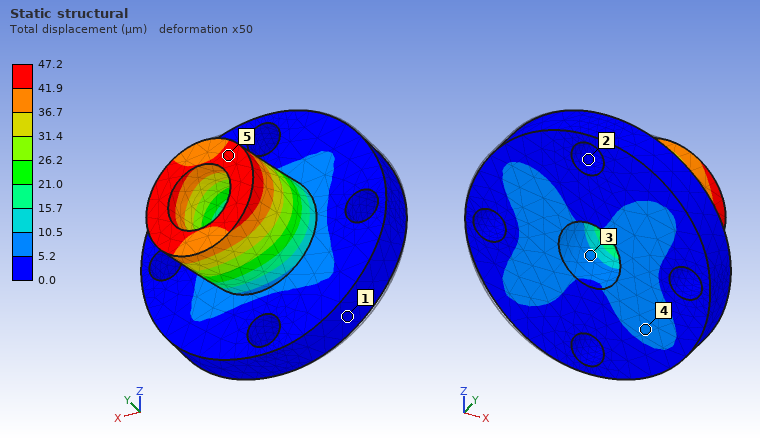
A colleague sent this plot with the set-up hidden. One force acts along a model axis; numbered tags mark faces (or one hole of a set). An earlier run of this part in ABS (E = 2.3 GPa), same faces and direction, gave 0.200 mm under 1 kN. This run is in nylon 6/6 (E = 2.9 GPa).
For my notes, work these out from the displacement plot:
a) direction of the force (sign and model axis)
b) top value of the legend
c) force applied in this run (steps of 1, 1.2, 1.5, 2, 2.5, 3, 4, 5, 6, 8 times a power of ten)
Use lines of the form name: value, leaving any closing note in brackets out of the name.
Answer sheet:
direction of the force: +X
top value of the legend: 47.2 µm
force applied in this run: 300 N
